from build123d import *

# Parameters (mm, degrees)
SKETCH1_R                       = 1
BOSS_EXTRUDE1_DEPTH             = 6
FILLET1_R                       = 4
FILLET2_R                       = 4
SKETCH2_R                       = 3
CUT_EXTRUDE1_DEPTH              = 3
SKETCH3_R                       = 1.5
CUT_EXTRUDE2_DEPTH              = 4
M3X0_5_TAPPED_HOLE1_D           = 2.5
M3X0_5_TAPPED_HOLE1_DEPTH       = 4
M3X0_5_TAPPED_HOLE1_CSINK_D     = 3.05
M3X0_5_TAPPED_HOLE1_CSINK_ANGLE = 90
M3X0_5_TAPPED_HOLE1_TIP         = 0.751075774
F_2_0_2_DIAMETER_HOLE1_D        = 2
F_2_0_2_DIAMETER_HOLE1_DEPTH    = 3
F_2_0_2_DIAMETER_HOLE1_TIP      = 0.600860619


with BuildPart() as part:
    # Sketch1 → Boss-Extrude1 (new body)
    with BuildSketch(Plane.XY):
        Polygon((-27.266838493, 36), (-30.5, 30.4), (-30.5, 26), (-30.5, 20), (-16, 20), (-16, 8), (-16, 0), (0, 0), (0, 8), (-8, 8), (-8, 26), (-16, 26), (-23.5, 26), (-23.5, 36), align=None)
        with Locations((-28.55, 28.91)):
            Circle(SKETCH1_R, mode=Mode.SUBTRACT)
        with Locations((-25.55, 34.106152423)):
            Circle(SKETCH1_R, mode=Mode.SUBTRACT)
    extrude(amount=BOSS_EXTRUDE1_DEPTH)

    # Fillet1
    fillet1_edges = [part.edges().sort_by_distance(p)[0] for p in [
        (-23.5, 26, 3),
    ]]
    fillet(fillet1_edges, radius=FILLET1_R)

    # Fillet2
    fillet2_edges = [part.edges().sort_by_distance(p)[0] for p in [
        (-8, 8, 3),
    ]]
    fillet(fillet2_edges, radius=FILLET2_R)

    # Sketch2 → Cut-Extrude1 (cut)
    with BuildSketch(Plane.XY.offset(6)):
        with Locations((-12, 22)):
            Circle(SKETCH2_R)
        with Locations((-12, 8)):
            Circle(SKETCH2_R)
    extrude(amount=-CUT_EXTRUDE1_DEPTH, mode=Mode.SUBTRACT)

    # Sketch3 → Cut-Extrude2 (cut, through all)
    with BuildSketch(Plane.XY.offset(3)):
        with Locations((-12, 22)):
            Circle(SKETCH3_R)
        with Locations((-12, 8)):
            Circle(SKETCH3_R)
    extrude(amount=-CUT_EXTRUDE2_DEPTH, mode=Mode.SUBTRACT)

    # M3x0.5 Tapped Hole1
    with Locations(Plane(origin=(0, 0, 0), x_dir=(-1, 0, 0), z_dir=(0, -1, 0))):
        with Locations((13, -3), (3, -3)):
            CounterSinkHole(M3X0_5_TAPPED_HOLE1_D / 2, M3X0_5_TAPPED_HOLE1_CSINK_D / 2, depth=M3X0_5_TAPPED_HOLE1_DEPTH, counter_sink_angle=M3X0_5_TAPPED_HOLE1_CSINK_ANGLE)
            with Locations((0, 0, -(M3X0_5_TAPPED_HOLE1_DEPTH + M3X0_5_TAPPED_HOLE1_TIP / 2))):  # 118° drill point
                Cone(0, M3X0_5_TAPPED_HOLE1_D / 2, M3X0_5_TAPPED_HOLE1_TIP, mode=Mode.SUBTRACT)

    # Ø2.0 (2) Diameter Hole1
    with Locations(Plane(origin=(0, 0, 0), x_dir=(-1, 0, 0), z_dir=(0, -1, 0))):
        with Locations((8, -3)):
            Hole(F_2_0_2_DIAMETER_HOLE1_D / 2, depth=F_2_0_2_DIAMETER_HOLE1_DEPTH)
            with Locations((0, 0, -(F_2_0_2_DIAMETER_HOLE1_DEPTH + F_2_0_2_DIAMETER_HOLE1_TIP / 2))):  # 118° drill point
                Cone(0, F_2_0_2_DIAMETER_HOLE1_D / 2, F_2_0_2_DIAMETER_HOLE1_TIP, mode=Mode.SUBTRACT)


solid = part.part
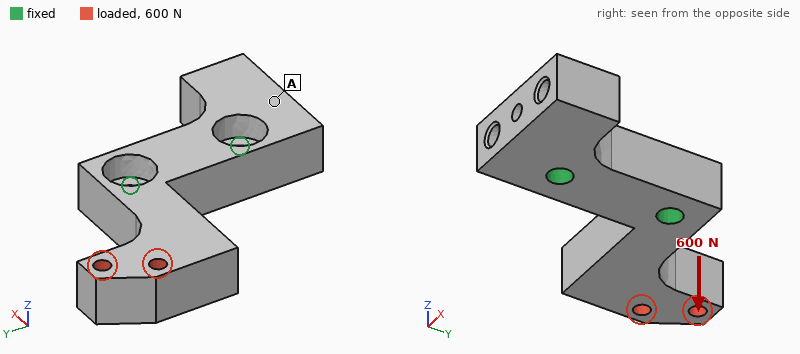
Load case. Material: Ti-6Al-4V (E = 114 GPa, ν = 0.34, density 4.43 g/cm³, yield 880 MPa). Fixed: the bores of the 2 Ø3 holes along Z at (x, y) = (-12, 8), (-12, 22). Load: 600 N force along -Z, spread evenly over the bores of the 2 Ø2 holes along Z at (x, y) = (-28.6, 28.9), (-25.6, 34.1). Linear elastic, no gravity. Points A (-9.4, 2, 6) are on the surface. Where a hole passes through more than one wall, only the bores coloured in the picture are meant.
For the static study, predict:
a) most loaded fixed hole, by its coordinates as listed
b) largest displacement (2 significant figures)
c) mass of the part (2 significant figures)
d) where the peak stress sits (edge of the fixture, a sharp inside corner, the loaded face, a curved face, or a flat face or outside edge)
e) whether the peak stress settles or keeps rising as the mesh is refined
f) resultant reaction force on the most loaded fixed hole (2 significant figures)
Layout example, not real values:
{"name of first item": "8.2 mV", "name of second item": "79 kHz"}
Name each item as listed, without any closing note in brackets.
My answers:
{"most loaded fixed hole, by its coordinates as listed": "(-12, 22)", "largest displacement": "0.22 mm", "mass of the part": "10 g", "where the peak stress sits": "edge of the fixture", "whether the peak stress settles or keeps rising as the mesh is refined": "keeps rising", "resultant reaction force on the most loaded fixed hole": "950 N"}
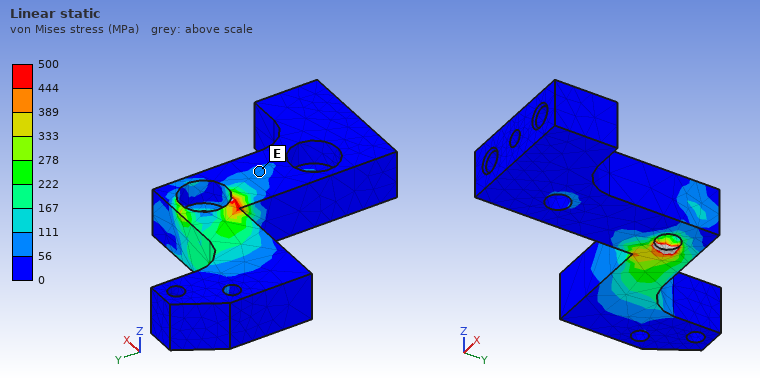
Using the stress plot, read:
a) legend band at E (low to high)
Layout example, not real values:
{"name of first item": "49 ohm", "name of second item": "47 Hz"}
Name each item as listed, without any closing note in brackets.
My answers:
{"legend band at E": "56 to 111 MPa"}
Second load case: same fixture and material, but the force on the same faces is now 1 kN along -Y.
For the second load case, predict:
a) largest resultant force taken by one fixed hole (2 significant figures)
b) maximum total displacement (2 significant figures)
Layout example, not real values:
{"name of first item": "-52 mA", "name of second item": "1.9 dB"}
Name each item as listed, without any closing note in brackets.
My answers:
{"largest resultant force taken by one fixed hole": "870 N", "maximum total displacement": "0.17 mm"}
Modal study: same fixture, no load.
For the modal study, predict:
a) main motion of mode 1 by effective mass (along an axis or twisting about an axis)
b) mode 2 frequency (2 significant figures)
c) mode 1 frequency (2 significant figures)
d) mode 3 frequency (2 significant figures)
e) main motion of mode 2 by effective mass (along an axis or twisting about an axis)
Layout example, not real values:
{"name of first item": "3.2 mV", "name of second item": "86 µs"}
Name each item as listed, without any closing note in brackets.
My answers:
{"main motion of mode 1 by effective mass": "along Z", "mode 2 frequency": "8100 Hz", "mode 1 frequency": "6600 Hz", "mode 3 frequency": "16 kHz", "main motion of mode 2 by effective mass": "along Y"}
